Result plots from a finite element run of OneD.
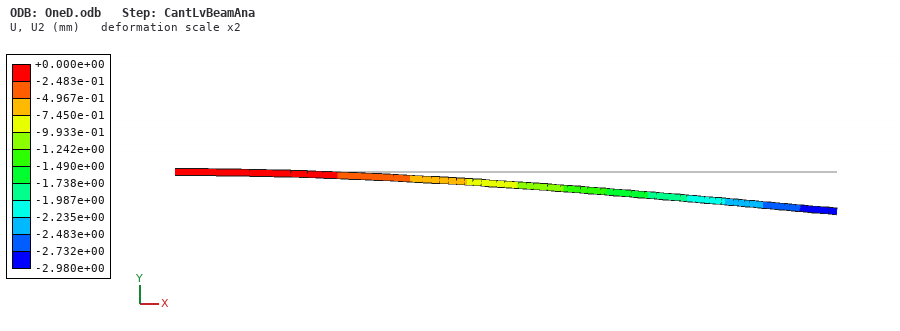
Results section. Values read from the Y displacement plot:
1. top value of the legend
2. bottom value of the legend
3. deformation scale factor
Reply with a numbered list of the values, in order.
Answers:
1. +0.000e+00 mm
2. -2.980e+00 mm
3. 2
